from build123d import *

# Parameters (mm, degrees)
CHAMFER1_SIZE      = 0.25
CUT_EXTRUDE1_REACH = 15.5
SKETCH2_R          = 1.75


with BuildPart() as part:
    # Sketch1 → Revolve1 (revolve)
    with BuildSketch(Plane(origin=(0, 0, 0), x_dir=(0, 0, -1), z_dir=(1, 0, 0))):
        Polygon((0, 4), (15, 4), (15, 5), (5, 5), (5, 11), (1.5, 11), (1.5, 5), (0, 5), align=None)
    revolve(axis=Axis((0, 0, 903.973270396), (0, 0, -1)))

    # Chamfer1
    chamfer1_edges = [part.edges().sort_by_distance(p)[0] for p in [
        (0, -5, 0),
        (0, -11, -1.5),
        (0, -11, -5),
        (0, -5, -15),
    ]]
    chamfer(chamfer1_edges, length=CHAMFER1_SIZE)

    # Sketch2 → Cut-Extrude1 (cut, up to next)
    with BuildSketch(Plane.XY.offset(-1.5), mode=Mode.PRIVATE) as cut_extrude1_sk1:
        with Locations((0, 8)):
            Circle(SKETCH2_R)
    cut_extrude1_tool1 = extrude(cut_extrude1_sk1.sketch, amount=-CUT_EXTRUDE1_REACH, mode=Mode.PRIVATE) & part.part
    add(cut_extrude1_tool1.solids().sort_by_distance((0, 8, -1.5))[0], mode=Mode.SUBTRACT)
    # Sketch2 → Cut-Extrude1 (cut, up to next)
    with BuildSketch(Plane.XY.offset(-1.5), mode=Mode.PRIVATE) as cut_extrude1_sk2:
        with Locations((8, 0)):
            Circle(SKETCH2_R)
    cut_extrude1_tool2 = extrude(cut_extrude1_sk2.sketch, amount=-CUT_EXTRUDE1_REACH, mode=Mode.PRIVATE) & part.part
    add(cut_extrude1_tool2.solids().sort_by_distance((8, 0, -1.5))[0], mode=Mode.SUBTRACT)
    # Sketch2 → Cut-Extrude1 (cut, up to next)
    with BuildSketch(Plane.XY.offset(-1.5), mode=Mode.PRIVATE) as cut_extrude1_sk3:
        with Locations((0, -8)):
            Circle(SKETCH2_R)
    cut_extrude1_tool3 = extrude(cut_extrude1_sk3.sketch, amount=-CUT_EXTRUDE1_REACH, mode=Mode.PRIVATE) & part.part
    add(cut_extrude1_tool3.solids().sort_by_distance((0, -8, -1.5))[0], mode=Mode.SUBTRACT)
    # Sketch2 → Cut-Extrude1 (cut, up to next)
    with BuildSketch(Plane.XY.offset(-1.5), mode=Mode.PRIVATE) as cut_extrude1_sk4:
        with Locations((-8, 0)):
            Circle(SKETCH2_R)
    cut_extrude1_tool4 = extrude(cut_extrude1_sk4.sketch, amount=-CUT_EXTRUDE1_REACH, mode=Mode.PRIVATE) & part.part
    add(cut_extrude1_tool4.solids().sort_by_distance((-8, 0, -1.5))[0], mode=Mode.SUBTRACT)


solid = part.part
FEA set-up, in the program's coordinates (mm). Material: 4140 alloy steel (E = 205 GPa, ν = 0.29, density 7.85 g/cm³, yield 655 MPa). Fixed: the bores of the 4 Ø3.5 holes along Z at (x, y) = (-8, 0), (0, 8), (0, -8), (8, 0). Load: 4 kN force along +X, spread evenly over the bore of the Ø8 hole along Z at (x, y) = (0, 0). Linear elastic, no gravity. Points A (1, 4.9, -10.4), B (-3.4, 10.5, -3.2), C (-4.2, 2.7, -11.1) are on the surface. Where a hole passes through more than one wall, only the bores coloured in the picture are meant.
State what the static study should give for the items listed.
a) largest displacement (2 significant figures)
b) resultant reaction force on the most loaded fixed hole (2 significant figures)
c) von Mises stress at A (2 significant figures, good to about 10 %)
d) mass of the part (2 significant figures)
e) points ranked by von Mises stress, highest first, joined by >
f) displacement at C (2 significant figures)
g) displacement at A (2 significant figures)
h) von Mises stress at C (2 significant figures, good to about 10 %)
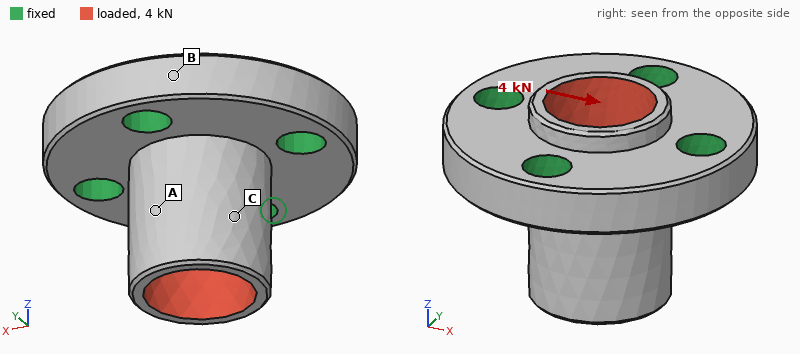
26 µm
1.7 kN
140 MPa
11 g
A > C > B
18 µm
15 µm
84 MPa
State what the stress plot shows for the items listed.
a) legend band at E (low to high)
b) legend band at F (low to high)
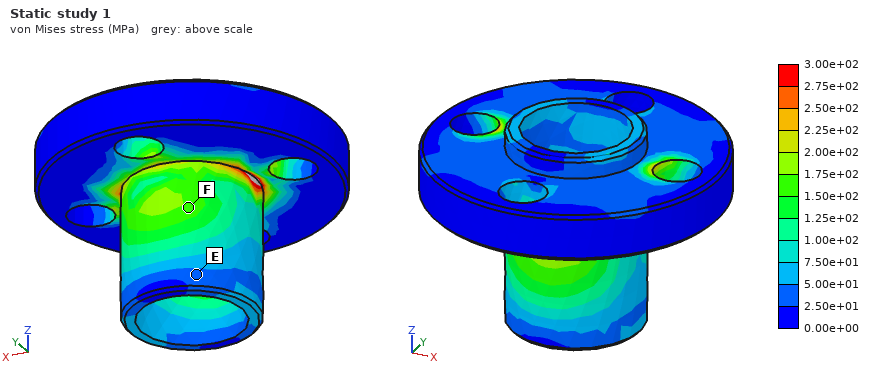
2.50e+01 to 5.00e+01 MPa
1.50e+02 to 1.75e+02 MPa
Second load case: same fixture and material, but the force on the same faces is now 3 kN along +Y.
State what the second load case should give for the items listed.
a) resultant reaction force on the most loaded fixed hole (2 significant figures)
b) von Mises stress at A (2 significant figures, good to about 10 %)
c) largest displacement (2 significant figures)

1.3 kN
52 MPa
19 µm
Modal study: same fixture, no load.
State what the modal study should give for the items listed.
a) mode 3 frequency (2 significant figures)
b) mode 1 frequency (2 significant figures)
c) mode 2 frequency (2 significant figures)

40 kHz
40 kHz
40 kHz
